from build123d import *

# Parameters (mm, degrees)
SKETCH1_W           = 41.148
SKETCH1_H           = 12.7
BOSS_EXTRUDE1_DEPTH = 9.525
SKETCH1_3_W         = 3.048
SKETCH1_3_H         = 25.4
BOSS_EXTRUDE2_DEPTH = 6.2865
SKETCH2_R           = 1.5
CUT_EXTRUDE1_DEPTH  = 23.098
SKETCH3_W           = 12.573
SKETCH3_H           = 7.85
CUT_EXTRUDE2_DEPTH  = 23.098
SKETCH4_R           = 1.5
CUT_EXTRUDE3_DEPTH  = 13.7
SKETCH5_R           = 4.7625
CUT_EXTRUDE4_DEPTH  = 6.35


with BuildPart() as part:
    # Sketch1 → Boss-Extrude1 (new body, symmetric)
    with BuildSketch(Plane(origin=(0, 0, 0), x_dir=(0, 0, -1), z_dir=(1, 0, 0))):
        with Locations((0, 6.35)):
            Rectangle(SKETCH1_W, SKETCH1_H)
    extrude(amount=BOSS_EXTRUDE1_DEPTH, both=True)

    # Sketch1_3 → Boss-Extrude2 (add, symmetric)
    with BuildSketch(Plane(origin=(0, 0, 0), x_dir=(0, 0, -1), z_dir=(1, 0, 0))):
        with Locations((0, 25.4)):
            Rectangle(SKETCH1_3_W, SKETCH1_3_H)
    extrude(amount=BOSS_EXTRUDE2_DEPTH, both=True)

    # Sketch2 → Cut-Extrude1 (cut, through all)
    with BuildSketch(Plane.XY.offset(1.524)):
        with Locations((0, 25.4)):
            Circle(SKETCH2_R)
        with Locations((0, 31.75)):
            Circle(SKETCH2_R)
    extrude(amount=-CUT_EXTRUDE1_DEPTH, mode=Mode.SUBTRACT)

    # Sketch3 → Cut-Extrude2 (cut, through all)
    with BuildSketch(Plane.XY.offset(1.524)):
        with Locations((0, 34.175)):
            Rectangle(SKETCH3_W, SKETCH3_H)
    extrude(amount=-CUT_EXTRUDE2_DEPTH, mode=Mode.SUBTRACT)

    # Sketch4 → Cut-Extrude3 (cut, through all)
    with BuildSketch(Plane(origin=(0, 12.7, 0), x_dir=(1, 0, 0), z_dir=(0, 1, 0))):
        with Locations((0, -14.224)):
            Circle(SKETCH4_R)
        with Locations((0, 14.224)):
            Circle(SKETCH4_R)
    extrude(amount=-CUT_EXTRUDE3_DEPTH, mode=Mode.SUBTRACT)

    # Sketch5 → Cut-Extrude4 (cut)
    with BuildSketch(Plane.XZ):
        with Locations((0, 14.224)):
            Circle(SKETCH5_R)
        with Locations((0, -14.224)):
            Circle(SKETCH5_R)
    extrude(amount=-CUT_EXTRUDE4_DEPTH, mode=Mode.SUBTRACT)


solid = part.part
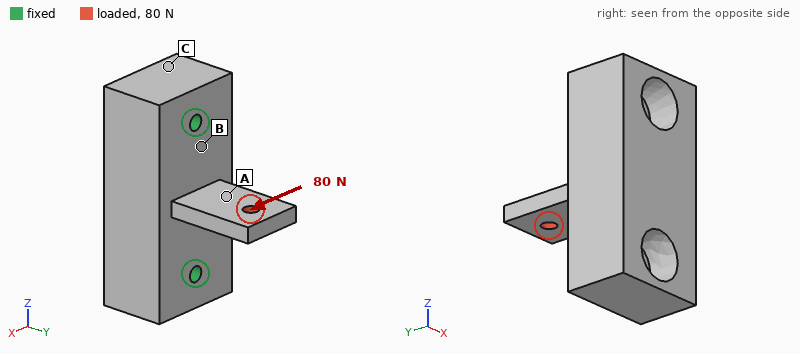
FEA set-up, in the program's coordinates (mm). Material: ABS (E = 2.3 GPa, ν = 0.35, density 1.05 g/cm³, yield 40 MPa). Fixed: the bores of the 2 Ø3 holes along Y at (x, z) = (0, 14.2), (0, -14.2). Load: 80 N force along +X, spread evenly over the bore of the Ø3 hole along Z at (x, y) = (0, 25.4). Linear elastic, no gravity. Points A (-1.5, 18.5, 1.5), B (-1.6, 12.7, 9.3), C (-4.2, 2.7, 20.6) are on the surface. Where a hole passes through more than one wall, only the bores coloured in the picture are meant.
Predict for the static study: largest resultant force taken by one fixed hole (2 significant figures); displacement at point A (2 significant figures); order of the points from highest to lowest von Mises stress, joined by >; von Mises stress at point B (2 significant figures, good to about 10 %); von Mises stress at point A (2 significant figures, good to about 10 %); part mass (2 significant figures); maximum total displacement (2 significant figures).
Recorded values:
40 N
0.082 mm
A > B > C
2.5 MPa
5.4 MPa
10 g
0.24 mm
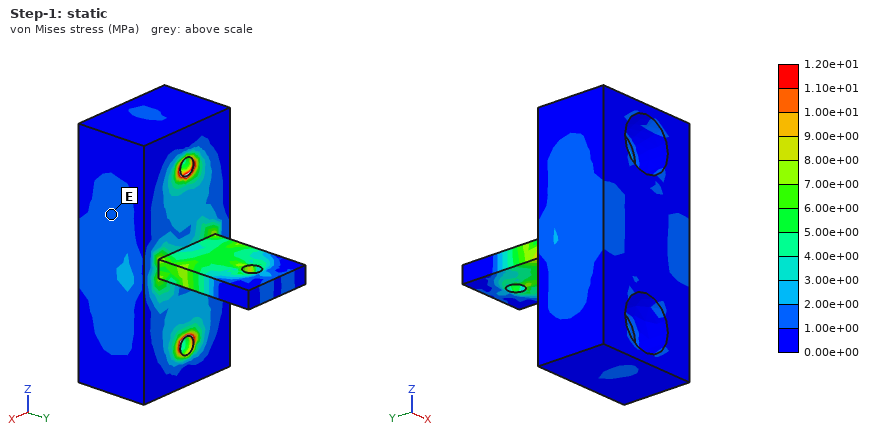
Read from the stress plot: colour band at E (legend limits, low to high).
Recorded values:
1.00e+00 to 2.00e+00 MPa
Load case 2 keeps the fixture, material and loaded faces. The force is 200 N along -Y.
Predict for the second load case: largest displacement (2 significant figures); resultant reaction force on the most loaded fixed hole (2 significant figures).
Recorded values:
69 µm
110 N
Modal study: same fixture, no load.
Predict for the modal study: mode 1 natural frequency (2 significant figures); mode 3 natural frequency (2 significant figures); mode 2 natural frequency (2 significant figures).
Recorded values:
2200 Hz
6100 Hz
3900 Hz
